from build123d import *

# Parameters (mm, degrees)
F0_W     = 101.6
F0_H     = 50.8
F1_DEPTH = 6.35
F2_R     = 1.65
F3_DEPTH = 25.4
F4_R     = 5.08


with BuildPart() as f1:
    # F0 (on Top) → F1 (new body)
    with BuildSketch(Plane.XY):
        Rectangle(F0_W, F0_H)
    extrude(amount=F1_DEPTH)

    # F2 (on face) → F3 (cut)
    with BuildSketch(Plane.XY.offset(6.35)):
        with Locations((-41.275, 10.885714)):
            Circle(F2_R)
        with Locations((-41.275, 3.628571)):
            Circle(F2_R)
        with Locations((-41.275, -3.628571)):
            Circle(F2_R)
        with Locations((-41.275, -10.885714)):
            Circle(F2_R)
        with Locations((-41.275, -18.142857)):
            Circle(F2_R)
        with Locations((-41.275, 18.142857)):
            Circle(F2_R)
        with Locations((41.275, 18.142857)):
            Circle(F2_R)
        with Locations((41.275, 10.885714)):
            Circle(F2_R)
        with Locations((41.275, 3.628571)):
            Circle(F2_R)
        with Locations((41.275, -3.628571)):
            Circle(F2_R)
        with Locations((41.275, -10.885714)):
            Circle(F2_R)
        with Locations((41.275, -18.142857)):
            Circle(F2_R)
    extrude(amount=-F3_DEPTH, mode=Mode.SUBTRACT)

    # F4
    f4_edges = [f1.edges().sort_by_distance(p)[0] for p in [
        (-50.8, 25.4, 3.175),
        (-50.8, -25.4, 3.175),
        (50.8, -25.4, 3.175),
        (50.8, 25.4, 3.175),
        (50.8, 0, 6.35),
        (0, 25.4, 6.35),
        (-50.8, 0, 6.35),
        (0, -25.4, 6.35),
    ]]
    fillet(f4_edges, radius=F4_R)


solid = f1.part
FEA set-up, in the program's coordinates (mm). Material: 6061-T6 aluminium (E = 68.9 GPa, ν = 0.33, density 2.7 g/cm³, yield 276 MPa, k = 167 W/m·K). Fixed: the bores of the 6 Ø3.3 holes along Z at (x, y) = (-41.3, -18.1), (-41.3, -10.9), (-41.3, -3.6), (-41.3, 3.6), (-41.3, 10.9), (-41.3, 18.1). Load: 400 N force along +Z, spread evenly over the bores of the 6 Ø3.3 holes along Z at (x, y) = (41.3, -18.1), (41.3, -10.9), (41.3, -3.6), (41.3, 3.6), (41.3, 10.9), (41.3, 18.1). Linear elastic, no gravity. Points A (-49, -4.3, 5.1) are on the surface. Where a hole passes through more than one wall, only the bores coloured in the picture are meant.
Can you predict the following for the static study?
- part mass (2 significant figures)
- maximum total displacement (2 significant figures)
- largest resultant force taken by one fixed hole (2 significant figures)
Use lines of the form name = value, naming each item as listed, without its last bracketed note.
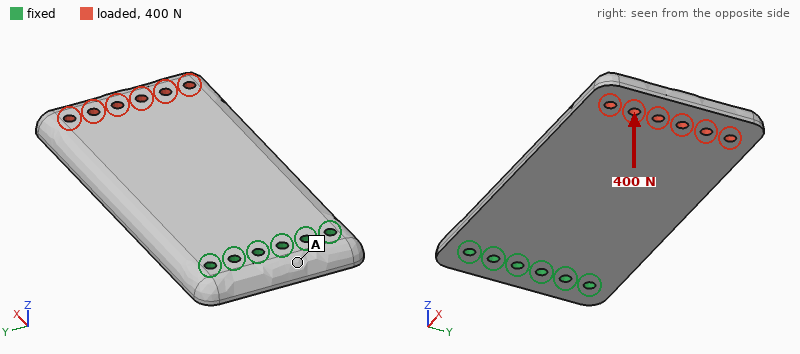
part mass = 82 g
maximum total displacement = 1.2 mm
largest resultant force taken by one fixed hole = 220 N
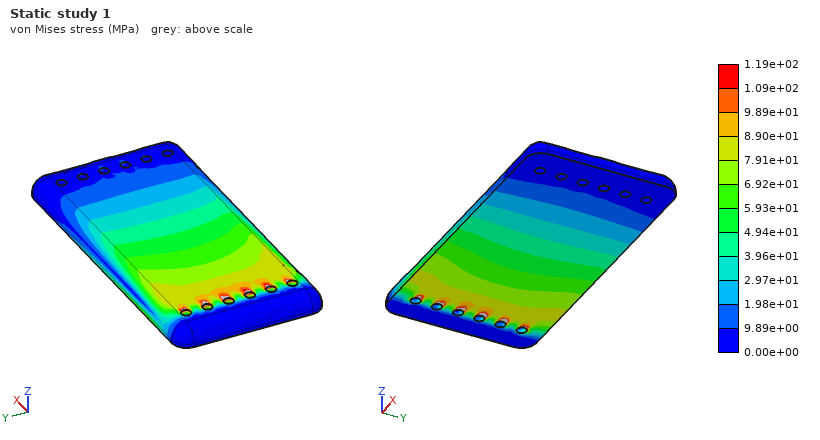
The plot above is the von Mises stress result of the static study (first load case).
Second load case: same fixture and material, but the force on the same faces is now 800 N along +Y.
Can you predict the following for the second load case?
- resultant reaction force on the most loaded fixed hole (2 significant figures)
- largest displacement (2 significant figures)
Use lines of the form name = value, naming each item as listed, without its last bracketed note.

resultant reaction force on the most loaded fixed hole = 1.4 kN
largest displacement = 55 µm
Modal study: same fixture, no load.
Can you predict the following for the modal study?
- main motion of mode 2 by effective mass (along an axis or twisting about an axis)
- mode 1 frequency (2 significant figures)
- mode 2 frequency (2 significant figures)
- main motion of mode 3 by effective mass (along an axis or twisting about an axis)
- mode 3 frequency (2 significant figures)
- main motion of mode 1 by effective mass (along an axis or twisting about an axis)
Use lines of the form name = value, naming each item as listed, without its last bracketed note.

main motion of mode 2 by effective mass = twisting about X
mode 1 frequency = 650 Hz
mode 2 frequency = 2400 Hz
main motion of mode 3 by effective mass = along Z
mode 3 frequency = 3900 Hz
main motion of mode 1 by effective mass = along Z
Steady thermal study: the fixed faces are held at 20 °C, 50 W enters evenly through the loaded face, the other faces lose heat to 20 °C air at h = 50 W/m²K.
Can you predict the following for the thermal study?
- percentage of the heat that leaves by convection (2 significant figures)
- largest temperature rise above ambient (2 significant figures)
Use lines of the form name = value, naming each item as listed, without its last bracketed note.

percentage of the heat that leaves by convection = 32 %
largest temperature rise above ambient = 62 K
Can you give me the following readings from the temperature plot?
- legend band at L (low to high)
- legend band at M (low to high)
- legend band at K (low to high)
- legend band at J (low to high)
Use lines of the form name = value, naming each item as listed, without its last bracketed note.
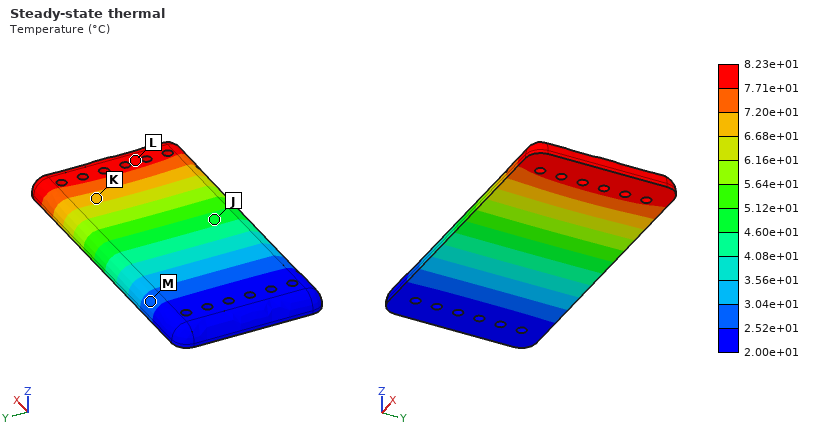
legend band at L = 7.71e+01 to 8.23e+01 °C
legend band at M = 2.52e+01 to 3.04e+01 °C
legend band at K = 6.68e+01 to 7.20e+01 °C
legend band at J = 4.60e+01 to 5.12e+01 °C
